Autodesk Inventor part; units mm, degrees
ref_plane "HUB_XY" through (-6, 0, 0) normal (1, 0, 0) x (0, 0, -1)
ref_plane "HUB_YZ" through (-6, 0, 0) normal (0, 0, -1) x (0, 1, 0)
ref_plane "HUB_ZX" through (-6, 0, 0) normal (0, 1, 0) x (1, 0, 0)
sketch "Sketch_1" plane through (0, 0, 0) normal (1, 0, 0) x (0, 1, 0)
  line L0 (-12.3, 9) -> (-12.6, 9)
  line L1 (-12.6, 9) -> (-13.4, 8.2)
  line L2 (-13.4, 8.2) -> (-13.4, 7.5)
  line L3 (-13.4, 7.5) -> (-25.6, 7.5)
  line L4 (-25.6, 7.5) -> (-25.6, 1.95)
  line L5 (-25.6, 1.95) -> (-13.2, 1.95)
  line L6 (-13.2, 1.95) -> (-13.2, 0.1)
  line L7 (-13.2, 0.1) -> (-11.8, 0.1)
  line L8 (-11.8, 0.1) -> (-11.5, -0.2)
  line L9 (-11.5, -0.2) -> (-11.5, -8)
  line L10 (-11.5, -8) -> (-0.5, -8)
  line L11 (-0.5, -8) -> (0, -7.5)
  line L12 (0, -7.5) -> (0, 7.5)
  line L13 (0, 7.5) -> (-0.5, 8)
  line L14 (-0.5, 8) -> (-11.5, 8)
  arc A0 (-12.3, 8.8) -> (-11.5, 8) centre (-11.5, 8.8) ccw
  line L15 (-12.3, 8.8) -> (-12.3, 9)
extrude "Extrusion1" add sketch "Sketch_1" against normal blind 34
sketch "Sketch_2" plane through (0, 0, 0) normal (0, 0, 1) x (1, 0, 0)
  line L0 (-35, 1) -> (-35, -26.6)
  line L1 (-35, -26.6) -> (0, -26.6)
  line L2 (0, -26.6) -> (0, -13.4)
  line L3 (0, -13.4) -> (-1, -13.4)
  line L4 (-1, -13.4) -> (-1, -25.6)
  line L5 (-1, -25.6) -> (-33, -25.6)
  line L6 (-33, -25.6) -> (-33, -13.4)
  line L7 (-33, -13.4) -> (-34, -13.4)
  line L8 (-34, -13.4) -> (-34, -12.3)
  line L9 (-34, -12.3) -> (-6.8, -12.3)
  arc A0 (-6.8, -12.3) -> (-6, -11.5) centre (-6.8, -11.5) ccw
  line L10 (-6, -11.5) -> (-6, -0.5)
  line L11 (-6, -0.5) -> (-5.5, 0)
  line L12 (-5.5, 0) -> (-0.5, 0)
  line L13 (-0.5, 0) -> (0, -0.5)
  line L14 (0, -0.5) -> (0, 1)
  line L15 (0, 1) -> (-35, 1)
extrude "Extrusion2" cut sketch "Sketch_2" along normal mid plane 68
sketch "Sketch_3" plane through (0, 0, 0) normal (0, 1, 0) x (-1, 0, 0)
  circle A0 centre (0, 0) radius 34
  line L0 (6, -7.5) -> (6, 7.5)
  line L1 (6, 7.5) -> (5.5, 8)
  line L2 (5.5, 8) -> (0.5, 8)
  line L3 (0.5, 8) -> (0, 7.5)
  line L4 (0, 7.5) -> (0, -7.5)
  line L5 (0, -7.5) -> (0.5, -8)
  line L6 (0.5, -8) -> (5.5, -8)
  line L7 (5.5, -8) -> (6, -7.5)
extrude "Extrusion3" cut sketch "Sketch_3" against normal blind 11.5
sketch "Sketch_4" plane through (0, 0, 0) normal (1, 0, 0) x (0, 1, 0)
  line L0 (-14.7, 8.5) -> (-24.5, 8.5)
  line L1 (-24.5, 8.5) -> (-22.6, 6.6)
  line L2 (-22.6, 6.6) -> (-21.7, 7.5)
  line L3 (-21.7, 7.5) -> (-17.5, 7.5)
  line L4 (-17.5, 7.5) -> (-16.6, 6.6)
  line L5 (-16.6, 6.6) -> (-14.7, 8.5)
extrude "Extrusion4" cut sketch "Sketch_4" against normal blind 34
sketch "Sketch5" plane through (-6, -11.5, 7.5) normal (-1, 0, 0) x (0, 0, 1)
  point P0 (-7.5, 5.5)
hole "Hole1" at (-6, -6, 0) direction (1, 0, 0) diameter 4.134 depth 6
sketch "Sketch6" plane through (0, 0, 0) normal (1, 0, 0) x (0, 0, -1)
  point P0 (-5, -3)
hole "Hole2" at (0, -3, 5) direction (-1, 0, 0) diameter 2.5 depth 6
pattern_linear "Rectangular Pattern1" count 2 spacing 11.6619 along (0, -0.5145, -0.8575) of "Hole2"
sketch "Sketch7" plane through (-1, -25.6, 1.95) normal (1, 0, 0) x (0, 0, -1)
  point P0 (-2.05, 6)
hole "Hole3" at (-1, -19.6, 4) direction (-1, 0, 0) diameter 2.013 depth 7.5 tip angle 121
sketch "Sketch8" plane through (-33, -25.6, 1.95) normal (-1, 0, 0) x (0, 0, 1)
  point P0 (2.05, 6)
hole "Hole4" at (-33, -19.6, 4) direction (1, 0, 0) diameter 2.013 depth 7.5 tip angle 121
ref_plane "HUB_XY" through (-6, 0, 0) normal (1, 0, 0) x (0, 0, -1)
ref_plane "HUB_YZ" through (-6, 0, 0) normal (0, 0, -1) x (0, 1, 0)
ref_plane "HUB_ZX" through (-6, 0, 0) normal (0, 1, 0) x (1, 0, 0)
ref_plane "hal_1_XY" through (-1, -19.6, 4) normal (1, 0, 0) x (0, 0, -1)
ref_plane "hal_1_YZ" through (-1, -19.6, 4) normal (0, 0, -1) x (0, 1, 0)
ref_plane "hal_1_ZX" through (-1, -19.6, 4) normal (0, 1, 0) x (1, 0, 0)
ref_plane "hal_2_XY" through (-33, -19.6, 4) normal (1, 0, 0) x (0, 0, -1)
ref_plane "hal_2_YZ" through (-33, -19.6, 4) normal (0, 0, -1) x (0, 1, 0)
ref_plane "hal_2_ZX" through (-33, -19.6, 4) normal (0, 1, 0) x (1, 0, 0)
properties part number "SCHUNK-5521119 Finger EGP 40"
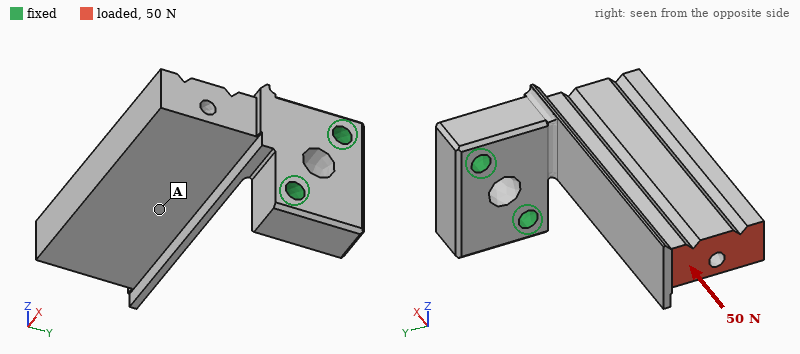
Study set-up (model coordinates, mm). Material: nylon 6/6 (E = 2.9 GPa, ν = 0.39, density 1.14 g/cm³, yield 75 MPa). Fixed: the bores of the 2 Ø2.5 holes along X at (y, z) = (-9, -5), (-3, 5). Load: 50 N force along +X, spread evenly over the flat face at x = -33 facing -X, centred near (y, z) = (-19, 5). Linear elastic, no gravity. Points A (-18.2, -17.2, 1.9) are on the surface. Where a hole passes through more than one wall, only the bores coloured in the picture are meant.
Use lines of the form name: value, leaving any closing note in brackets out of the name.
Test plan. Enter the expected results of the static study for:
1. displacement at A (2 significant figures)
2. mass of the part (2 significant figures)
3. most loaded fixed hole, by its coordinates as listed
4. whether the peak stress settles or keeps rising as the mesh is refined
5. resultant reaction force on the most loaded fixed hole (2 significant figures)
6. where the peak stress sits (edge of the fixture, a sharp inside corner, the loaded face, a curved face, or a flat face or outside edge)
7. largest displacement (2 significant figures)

displacement at A: 0.26 mm
mass of the part: 3.8 g
most loaded fixed hole, by its coordinates as listed: (-9, -5)
whether the peak stress settles or keeps rising as the mesh is refined: keeps rising
resultant reaction force on the most loaded fixed hole: 34 N
where the peak stress sits: a sharp inside corner
largest displacement: 0.53 mm
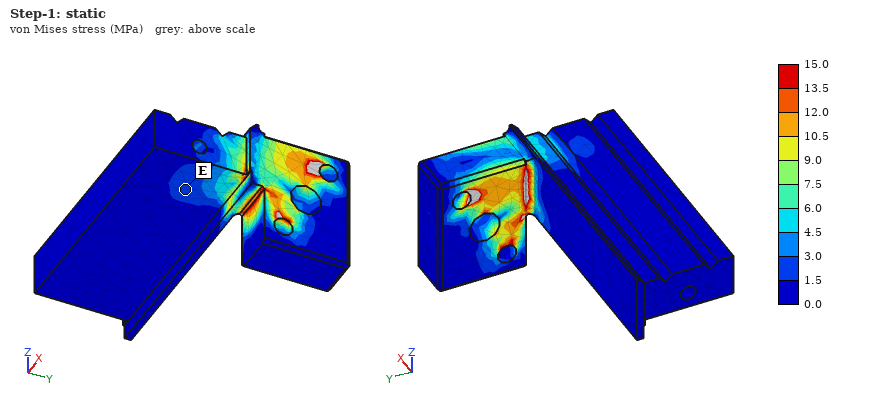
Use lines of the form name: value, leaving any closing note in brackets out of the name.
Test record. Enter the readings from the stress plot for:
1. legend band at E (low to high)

legend band at E: 1.5 to 3.0 MPa
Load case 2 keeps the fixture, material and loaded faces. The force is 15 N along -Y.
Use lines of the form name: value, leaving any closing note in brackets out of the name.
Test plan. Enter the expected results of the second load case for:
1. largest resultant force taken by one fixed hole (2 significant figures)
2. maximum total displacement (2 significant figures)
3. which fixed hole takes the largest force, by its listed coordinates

largest resultant force taken by one fixed hole: 22 N
maximum total displacement: 0.53 mm
which fixed hole takes the largest force, by its listed coordinates: (-3, 5)
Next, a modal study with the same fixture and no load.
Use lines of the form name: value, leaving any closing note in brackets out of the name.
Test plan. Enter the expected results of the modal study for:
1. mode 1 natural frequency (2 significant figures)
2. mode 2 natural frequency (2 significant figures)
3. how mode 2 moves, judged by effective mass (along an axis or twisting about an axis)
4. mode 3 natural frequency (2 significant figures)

mode 1 natural frequency: 870 Hz
mode 2 natural frequency: 1000 Hz
how mode 2 moves, judged by effective mass: along Z
mode 3 natural frequency: 3000 Hz
